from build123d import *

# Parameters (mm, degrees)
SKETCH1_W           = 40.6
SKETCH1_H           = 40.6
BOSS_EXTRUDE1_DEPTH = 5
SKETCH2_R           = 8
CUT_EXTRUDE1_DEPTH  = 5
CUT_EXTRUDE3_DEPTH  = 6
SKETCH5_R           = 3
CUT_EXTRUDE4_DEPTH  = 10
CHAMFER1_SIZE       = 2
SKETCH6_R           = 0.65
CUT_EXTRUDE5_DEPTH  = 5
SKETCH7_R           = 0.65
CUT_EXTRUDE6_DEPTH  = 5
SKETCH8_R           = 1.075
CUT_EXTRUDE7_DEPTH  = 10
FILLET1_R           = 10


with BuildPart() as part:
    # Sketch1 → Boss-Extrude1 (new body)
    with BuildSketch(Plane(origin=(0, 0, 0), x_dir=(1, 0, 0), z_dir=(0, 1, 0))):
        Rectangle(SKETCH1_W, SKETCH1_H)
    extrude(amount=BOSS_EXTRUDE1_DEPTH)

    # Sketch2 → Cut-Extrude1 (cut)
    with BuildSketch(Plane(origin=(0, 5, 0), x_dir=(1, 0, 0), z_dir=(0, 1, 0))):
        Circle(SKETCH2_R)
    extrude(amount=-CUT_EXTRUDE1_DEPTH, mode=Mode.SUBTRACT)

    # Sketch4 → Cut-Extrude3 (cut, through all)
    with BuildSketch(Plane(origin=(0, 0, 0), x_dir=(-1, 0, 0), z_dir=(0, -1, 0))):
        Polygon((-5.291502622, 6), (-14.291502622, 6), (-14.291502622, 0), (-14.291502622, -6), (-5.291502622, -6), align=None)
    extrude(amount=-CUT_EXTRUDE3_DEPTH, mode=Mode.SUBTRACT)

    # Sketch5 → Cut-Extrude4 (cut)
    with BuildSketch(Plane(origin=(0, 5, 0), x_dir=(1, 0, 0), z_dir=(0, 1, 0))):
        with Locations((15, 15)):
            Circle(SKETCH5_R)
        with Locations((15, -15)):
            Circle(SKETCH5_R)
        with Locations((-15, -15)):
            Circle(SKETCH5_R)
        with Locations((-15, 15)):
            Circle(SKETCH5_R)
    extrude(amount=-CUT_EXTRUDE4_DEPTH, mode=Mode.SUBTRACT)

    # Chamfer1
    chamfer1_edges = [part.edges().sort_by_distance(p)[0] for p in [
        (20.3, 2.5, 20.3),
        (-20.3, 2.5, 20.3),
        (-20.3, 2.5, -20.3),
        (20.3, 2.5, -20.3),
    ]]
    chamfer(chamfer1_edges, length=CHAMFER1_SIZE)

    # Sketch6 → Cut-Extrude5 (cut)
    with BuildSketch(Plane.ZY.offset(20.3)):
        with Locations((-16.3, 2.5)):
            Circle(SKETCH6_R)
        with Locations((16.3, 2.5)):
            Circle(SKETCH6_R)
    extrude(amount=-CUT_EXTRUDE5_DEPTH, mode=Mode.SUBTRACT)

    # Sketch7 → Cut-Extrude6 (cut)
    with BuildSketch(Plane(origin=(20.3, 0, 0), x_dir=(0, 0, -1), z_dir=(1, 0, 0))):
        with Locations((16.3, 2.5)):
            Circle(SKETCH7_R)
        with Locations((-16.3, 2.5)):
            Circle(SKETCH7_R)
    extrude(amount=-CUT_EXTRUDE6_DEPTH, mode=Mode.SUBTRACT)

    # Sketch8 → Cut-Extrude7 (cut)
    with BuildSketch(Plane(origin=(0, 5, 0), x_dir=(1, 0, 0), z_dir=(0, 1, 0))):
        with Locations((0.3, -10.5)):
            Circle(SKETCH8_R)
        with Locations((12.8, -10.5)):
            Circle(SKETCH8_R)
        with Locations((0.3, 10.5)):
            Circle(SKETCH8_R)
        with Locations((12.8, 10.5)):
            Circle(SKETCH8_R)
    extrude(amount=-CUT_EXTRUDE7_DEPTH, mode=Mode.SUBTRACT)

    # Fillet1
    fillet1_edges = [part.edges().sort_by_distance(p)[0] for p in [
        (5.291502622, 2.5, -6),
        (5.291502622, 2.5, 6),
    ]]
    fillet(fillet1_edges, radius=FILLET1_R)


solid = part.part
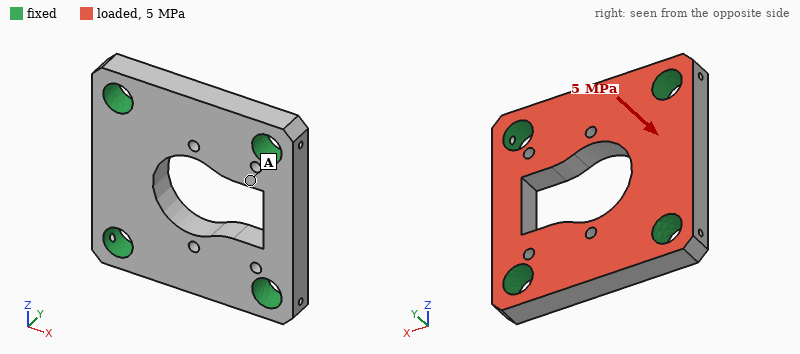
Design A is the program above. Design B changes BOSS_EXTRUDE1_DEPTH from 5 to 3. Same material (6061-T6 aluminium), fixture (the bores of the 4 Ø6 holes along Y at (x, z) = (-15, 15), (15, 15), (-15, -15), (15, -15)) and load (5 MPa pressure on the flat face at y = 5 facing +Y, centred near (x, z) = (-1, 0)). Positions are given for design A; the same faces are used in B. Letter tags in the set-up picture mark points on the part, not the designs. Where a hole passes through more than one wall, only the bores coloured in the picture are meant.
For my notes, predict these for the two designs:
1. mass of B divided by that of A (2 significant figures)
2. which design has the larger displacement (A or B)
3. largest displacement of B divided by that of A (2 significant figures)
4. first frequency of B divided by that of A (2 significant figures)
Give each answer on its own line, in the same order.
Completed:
0.60
B
3.6
0.70
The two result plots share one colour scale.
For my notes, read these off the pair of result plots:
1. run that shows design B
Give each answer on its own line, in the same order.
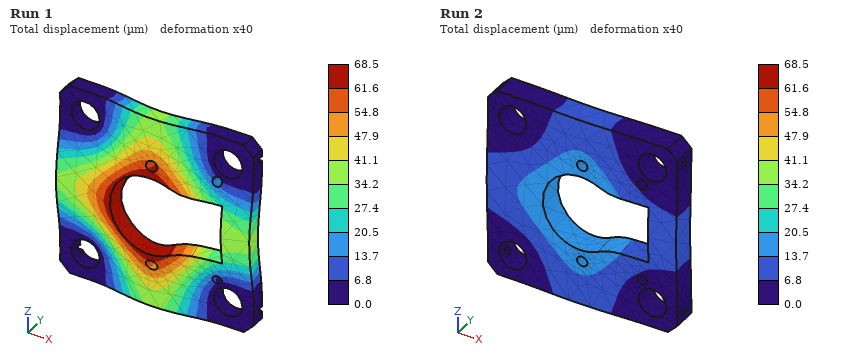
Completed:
Run 1
